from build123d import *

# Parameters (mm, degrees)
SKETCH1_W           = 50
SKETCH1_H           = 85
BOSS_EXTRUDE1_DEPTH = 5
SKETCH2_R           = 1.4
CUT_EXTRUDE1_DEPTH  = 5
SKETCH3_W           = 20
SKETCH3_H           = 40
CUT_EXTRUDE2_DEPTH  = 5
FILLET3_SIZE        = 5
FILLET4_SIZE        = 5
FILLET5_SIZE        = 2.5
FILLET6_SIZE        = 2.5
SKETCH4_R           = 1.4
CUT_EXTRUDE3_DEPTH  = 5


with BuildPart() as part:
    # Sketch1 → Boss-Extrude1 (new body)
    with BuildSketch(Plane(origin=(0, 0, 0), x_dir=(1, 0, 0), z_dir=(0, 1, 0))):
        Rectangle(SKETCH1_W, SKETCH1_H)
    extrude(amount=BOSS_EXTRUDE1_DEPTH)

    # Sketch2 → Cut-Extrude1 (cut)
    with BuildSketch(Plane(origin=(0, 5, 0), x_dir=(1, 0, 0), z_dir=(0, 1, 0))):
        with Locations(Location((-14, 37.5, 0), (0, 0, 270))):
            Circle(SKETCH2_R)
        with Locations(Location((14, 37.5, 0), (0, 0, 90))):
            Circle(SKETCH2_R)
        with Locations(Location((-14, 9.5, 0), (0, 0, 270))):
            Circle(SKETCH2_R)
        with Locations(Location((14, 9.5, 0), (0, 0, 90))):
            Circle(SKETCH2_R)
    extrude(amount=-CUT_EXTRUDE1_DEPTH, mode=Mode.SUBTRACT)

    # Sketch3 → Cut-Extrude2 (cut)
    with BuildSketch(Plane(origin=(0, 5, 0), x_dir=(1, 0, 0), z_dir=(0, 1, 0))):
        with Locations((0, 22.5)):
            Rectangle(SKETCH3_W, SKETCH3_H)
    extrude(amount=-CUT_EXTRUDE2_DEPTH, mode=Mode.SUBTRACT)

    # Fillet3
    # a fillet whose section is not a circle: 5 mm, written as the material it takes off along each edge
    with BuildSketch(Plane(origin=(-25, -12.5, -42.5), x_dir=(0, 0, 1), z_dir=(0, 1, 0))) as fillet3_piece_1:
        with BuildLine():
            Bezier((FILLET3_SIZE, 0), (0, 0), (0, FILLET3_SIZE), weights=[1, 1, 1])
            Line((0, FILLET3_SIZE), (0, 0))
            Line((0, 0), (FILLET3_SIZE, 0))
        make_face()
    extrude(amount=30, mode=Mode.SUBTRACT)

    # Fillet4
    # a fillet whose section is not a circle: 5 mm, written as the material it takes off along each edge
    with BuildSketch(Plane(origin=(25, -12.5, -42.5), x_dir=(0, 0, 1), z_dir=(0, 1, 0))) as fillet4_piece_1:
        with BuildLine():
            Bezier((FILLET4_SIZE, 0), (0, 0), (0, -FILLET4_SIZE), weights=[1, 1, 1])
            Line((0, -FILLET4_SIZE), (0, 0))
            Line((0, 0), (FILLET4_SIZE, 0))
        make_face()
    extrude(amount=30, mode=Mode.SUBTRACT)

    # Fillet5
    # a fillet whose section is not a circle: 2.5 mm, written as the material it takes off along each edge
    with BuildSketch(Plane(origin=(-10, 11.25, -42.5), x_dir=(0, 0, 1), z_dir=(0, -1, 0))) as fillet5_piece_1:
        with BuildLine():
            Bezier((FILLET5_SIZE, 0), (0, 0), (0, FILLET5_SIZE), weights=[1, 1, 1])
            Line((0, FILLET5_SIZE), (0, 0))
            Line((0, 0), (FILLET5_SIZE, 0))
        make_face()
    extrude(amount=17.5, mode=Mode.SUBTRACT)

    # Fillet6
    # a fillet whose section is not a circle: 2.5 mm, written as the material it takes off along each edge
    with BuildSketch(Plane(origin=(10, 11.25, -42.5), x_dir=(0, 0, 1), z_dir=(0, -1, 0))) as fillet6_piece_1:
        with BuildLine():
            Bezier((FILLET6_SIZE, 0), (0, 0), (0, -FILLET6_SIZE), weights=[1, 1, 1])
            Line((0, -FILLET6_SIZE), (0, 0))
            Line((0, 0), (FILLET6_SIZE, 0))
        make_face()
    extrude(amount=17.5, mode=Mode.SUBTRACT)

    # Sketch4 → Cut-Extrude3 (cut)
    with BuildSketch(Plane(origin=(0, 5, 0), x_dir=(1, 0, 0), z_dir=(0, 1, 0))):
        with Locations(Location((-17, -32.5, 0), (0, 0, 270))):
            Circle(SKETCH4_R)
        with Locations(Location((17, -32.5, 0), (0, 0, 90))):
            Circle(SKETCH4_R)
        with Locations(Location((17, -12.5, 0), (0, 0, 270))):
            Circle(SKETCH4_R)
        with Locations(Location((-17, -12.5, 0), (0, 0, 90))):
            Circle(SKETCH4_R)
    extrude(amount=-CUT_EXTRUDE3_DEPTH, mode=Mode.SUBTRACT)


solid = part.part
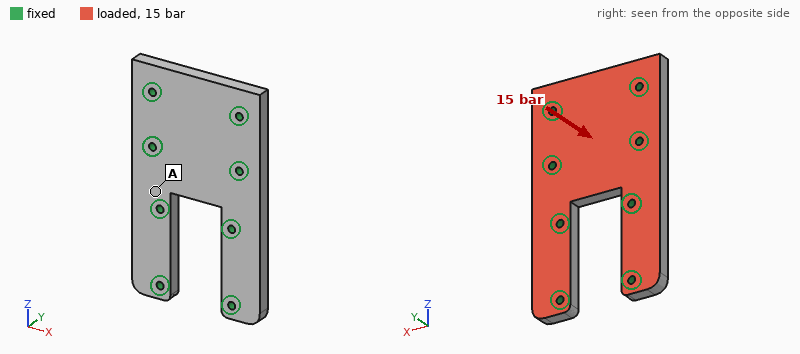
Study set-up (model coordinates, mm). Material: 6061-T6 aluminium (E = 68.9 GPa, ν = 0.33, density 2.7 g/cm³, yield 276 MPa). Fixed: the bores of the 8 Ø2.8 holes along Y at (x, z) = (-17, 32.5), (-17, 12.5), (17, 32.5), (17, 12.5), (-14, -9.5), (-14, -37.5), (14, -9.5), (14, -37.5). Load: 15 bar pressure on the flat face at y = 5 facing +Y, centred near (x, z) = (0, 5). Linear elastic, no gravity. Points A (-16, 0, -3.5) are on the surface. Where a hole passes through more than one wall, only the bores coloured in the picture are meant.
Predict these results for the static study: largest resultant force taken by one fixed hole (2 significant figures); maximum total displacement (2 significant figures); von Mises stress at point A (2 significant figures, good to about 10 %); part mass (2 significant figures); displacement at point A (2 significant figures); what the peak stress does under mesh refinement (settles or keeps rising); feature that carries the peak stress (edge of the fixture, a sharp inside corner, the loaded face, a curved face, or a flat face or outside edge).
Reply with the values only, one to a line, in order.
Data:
750 N
15 µm
16 MPa
46 g
2.7 µm
keeps rising
edge of the fixture
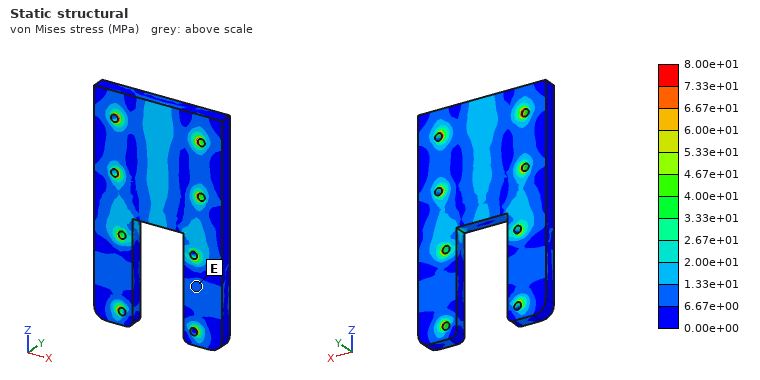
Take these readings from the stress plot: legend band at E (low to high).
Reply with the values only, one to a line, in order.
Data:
6.67e+00 to 1.33e+01 MPa
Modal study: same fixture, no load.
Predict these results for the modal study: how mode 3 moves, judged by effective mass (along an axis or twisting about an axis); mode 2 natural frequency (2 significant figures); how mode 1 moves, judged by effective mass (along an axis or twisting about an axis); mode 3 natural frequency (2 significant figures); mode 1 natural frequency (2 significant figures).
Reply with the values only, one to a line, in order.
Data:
twisting about Z
19 kHz
along Y
20 kHz
17 kHz
